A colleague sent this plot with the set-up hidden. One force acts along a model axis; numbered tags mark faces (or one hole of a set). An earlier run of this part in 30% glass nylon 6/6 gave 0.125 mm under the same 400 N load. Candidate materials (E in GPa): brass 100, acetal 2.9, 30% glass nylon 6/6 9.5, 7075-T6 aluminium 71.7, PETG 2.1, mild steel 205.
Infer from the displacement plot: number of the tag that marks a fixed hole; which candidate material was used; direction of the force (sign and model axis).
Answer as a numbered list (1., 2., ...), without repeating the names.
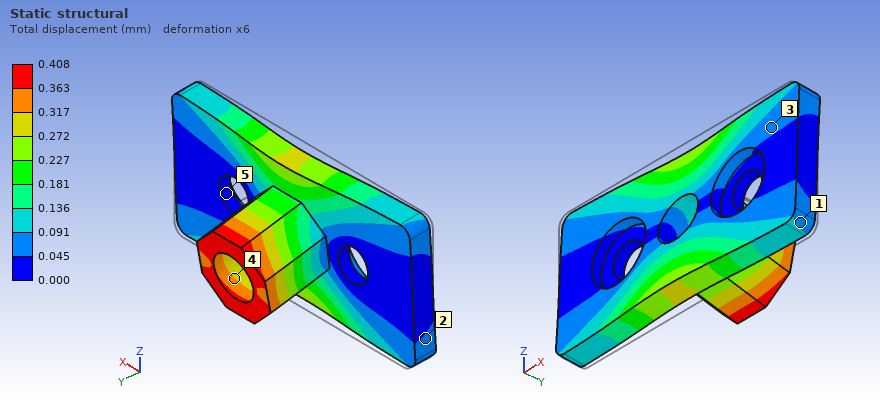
1. 5
2. acetal
3. -Z
